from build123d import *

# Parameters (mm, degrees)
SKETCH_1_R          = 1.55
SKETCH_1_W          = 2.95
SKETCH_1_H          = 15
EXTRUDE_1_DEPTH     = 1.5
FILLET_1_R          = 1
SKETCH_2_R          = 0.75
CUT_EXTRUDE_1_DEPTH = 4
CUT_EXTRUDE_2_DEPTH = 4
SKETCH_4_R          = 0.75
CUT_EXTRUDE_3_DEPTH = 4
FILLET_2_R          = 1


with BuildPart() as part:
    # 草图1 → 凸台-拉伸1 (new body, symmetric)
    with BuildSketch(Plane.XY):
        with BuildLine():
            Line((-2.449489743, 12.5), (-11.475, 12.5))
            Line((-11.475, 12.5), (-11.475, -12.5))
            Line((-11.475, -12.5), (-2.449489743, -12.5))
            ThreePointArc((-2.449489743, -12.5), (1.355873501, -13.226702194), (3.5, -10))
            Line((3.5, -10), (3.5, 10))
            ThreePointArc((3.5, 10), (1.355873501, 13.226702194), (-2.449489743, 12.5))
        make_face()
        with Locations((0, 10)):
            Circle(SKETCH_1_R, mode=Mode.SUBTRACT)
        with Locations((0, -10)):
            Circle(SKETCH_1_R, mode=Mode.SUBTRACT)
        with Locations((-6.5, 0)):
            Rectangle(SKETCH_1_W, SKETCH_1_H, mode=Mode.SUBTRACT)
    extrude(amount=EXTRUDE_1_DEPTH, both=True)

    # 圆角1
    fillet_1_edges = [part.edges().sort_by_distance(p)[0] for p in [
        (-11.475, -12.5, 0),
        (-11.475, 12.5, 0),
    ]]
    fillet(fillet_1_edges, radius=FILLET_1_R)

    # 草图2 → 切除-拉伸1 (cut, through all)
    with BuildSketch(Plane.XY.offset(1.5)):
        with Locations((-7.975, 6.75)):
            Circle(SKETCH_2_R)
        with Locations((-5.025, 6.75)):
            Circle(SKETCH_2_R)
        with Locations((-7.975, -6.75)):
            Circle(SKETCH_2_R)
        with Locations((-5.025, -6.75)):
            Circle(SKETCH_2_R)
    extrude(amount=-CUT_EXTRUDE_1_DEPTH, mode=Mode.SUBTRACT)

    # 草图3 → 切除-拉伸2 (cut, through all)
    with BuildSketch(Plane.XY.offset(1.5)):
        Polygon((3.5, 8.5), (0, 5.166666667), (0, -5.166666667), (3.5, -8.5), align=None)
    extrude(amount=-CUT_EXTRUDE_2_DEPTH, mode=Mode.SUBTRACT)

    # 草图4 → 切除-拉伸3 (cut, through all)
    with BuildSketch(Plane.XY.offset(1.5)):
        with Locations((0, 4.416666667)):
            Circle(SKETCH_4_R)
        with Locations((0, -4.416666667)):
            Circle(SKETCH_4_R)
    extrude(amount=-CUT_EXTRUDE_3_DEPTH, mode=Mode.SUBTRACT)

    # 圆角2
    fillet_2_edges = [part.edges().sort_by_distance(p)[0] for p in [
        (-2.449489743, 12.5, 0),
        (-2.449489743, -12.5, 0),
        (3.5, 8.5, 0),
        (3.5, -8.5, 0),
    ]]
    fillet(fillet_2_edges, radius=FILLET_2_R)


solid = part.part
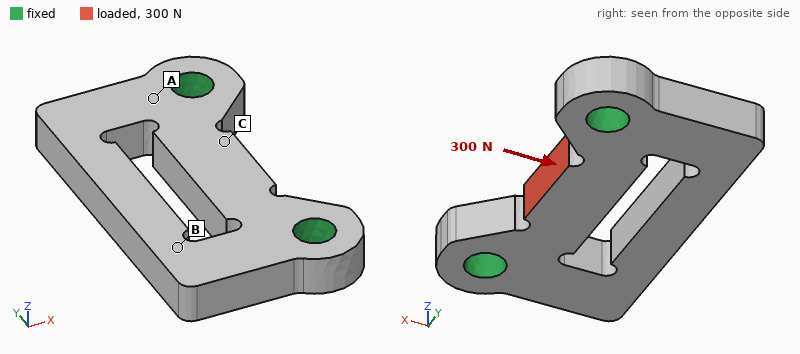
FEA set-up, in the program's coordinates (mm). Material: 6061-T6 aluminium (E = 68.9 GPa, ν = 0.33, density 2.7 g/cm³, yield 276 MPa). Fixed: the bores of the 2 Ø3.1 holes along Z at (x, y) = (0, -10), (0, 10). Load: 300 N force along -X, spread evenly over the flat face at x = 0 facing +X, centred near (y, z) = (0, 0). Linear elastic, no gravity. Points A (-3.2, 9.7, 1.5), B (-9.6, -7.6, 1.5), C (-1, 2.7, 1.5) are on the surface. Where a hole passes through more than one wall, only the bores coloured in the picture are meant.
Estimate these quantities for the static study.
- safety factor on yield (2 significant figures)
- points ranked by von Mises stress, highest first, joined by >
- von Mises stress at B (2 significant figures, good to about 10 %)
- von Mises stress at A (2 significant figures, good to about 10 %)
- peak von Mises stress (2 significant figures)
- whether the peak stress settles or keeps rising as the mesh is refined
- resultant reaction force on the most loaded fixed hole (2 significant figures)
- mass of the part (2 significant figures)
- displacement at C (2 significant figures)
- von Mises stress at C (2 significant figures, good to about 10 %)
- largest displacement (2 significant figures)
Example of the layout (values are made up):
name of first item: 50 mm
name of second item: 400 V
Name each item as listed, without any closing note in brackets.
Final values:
safety factor on yield: 4.9
points ranked by von Mises stress, highest first, joined by >: C > A > B
von Mises stress at B: 3.2 MPa
von Mises stress at A: 8.6 MPa
peak von Mises stress: 56 MPa
whether the peak stress settles or keeps rising as the mesh is refined: settles
resultant reaction force on the most loaded fixed hole: 170 N
mass of the part: 2.2 g
displacement at C: 4.8 µm
von Mises stress at C: 16 MPa
largest displacement: 6.0 µm
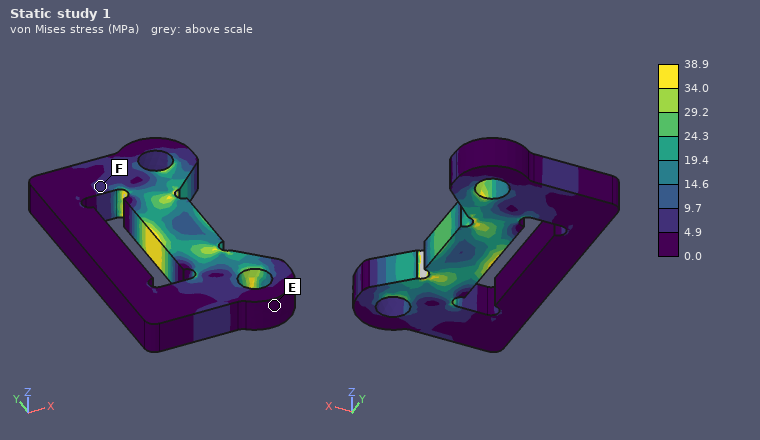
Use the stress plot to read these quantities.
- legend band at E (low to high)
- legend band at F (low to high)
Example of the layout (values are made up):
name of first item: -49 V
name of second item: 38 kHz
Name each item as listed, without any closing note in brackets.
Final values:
legend band at E: 0.0 to 4.9 MPa
legend band at F: 4.9 to 9.7 MPa
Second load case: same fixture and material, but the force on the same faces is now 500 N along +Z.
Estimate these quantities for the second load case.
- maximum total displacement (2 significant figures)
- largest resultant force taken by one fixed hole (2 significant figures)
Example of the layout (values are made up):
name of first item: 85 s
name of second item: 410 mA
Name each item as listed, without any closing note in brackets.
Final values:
maximum total displacement: 39 µm
largest resultant force taken by one fixed hole: 250 N
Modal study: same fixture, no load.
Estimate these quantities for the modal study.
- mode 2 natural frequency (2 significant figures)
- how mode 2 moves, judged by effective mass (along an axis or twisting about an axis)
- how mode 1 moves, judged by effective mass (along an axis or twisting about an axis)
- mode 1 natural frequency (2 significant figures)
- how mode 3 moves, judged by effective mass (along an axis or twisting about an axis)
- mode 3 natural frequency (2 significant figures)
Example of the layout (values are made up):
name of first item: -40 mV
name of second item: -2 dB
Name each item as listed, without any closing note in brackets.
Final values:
mode 2 natural frequency: 24 kHz
how mode 2 moves, judged by effective mass: twisting about X
how mode 1 moves, judged by effective mass: along Z
mode 1 natural frequency: 14 kHz
how mode 3 moves, judged by effective mass: along Y
mode 3 natural frequency: 28 kHz
